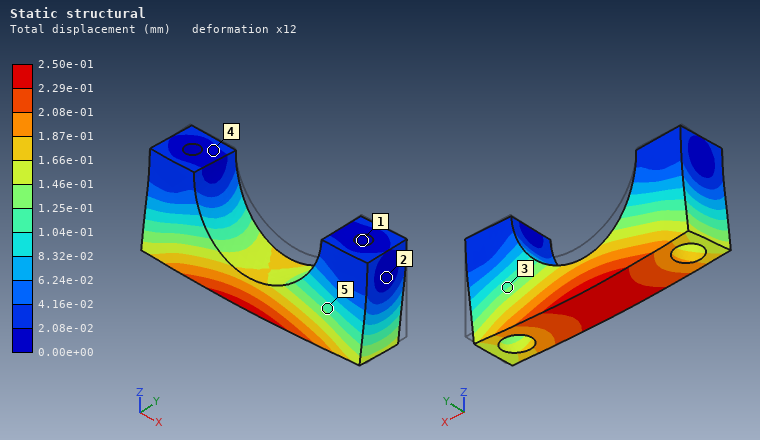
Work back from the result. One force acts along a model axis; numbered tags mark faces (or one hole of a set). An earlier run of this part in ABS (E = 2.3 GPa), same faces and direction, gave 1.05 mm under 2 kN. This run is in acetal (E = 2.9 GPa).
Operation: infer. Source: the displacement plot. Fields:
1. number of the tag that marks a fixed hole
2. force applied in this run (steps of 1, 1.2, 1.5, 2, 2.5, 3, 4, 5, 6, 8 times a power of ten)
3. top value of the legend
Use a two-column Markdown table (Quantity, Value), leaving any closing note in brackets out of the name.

| Quantity | Value |
|---|---|
| number of the tag that marks a fixed hole | 1 |
| force applied in this run | 600 N |
| top value of the legend | 2.50e-01 mm |
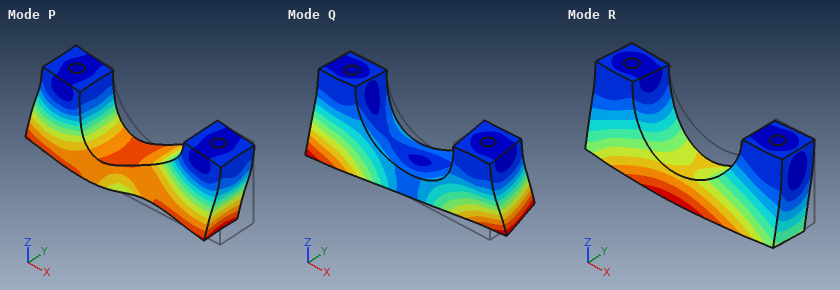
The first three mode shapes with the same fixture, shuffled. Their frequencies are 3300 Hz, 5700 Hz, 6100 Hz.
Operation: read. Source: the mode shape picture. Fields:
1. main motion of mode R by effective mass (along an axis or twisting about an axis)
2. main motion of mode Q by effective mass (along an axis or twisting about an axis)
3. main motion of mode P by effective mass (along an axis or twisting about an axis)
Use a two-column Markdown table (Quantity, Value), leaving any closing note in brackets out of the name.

| Quantity | Value |
|---|---|
| main motion of mode R by effective mass | along Y |
| main motion of mode Q by effective mass | twisting about Z |
| main motion of mode P by effective mass | along X |
